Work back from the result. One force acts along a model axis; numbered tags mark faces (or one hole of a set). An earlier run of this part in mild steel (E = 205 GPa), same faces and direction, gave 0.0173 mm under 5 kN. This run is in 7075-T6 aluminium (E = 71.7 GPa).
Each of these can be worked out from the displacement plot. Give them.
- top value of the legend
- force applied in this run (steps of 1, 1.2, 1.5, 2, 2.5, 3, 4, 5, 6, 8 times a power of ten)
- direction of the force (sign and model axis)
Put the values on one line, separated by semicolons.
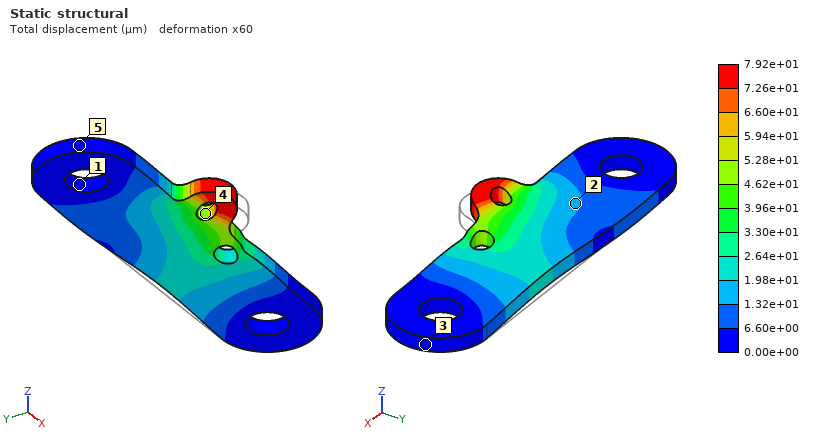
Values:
7.92e+01 µm; 8 kN; -X
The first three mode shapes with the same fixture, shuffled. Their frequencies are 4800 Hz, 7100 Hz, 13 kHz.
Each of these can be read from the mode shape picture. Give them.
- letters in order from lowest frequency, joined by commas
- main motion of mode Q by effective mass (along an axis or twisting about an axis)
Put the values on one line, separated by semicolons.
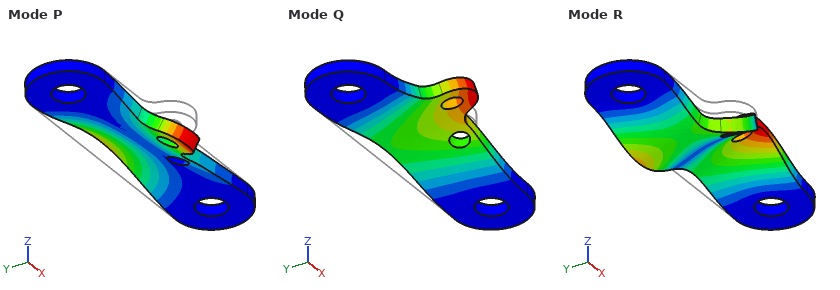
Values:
Q, P, R; along Z
